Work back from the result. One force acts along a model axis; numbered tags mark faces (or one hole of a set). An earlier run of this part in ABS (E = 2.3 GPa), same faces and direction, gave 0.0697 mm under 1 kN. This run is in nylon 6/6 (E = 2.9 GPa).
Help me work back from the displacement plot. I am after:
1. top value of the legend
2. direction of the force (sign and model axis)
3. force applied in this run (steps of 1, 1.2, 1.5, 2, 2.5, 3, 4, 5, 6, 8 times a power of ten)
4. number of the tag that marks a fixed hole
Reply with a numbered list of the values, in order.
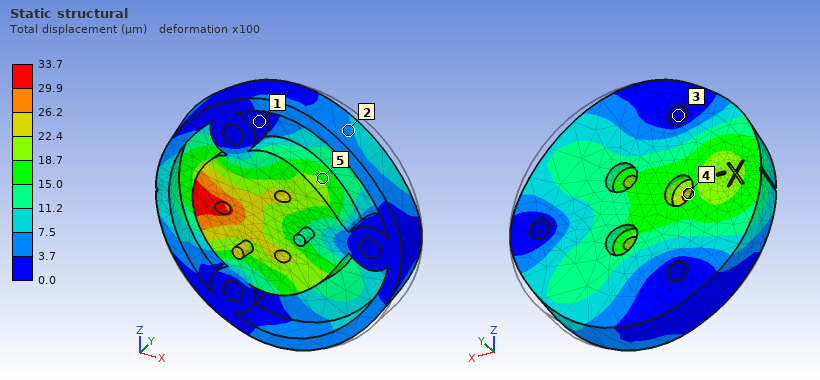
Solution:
1. 33.7 µm
2. -X
3. 600 N
4. 3
